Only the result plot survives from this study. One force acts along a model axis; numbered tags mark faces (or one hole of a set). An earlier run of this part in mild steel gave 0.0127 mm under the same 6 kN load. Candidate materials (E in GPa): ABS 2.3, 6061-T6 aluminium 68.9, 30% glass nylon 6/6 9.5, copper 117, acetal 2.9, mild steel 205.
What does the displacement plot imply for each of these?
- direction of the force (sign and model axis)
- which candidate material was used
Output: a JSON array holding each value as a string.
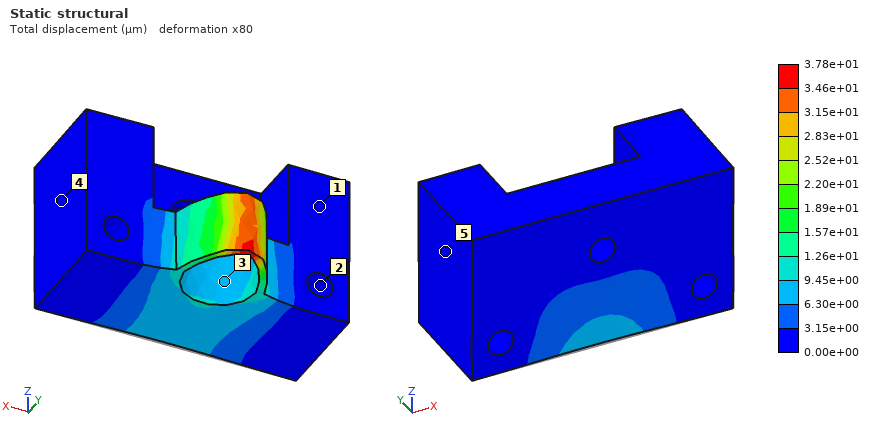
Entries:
["+Y", "6061-T6 aluminium"]
